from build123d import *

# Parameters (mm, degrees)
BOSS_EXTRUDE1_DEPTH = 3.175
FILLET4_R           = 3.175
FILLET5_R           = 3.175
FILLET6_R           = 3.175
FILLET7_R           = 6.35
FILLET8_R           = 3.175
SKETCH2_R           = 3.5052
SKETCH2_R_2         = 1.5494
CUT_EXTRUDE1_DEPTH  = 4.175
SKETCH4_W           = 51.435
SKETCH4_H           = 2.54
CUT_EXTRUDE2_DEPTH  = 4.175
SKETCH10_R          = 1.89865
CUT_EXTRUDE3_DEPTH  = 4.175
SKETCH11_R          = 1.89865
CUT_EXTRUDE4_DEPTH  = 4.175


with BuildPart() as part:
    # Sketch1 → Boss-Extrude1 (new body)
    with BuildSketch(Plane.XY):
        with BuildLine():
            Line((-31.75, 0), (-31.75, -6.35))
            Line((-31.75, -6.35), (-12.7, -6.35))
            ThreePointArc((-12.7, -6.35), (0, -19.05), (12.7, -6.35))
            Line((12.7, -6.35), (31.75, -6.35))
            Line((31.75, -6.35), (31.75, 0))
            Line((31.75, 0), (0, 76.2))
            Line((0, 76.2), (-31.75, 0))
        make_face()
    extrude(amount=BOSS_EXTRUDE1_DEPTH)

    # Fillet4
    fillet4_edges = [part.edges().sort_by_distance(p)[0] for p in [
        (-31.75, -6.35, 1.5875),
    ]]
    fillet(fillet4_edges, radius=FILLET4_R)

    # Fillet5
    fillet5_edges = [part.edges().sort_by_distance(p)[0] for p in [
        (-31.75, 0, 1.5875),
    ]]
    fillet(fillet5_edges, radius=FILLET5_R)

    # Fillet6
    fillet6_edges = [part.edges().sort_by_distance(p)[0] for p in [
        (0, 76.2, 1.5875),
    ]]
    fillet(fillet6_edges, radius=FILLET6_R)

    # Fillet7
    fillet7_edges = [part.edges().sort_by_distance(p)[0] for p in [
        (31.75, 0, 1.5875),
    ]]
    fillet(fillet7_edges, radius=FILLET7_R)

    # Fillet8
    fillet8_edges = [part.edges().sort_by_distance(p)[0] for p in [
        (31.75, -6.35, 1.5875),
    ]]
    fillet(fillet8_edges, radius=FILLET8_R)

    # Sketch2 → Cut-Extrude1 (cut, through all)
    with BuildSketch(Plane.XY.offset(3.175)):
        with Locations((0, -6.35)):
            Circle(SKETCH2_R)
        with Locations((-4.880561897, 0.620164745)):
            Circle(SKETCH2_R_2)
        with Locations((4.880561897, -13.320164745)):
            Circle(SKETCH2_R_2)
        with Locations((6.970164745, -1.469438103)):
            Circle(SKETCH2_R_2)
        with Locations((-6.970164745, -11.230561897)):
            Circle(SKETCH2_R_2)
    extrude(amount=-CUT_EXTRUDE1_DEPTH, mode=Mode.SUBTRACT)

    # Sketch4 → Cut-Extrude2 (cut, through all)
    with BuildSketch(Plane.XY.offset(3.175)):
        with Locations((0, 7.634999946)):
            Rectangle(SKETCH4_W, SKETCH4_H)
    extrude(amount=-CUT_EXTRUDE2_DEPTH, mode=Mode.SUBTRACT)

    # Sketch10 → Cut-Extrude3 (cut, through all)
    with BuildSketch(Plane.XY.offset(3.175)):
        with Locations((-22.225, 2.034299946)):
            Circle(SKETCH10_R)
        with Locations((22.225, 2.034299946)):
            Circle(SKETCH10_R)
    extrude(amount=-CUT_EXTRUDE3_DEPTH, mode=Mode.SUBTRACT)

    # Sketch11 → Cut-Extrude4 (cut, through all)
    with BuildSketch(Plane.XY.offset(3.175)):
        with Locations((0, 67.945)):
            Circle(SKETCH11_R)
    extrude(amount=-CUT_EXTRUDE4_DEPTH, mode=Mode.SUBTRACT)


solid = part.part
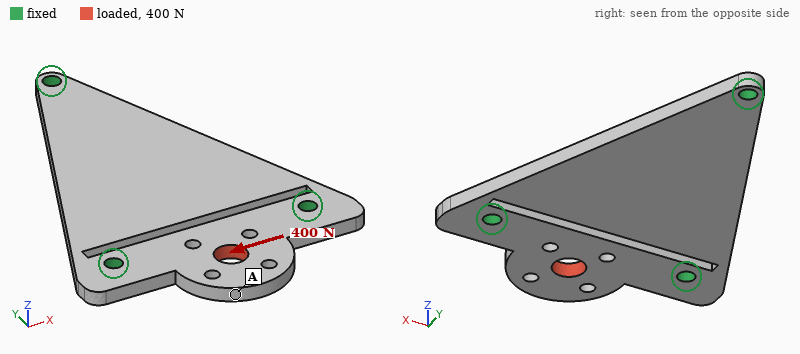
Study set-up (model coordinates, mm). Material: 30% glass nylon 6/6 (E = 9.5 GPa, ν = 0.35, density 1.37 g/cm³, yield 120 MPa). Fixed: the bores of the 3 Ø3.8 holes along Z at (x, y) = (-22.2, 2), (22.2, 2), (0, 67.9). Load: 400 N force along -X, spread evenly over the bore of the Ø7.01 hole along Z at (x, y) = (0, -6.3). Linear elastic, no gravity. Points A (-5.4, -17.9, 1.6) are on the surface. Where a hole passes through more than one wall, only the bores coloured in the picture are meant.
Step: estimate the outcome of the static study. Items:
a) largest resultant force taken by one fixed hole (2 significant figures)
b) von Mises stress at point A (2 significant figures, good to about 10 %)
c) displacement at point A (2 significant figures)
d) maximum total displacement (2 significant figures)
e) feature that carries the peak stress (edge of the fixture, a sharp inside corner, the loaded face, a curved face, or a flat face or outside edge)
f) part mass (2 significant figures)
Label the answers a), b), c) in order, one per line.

a) 210 N
b) 1.7 MPa
c) 18 µm
d) 22 µm
e) a curved face
f) 12 g
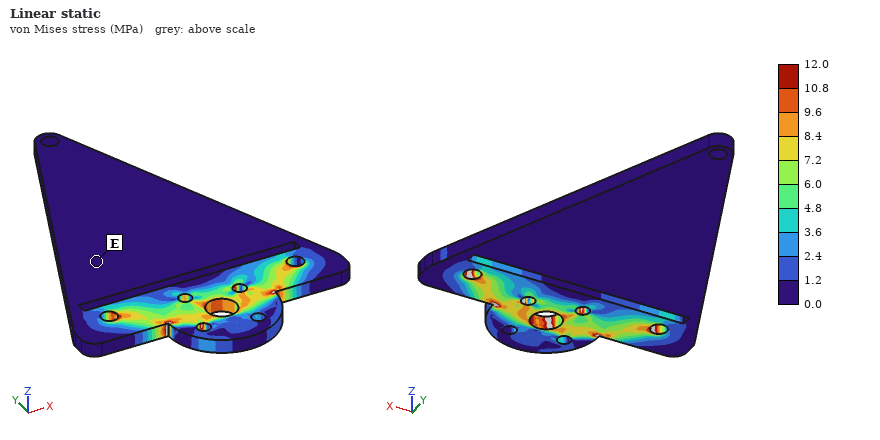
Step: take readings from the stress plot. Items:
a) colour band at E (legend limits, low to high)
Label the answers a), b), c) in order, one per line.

a) 0.0 to 1.2 MPa
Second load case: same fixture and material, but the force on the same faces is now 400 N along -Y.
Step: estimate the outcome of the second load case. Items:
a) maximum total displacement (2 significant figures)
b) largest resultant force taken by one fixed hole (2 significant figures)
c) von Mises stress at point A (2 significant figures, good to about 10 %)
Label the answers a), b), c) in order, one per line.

a) 56 µm
b) 230 N
c) 4.8 MPa
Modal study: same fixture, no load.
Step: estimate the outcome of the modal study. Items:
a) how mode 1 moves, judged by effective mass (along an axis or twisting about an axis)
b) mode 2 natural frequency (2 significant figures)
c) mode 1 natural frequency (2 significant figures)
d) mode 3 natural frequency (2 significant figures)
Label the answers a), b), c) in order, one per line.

a) along Z
b) 2400 Hz
c) 1200 Hz
d) 2400 Hz
